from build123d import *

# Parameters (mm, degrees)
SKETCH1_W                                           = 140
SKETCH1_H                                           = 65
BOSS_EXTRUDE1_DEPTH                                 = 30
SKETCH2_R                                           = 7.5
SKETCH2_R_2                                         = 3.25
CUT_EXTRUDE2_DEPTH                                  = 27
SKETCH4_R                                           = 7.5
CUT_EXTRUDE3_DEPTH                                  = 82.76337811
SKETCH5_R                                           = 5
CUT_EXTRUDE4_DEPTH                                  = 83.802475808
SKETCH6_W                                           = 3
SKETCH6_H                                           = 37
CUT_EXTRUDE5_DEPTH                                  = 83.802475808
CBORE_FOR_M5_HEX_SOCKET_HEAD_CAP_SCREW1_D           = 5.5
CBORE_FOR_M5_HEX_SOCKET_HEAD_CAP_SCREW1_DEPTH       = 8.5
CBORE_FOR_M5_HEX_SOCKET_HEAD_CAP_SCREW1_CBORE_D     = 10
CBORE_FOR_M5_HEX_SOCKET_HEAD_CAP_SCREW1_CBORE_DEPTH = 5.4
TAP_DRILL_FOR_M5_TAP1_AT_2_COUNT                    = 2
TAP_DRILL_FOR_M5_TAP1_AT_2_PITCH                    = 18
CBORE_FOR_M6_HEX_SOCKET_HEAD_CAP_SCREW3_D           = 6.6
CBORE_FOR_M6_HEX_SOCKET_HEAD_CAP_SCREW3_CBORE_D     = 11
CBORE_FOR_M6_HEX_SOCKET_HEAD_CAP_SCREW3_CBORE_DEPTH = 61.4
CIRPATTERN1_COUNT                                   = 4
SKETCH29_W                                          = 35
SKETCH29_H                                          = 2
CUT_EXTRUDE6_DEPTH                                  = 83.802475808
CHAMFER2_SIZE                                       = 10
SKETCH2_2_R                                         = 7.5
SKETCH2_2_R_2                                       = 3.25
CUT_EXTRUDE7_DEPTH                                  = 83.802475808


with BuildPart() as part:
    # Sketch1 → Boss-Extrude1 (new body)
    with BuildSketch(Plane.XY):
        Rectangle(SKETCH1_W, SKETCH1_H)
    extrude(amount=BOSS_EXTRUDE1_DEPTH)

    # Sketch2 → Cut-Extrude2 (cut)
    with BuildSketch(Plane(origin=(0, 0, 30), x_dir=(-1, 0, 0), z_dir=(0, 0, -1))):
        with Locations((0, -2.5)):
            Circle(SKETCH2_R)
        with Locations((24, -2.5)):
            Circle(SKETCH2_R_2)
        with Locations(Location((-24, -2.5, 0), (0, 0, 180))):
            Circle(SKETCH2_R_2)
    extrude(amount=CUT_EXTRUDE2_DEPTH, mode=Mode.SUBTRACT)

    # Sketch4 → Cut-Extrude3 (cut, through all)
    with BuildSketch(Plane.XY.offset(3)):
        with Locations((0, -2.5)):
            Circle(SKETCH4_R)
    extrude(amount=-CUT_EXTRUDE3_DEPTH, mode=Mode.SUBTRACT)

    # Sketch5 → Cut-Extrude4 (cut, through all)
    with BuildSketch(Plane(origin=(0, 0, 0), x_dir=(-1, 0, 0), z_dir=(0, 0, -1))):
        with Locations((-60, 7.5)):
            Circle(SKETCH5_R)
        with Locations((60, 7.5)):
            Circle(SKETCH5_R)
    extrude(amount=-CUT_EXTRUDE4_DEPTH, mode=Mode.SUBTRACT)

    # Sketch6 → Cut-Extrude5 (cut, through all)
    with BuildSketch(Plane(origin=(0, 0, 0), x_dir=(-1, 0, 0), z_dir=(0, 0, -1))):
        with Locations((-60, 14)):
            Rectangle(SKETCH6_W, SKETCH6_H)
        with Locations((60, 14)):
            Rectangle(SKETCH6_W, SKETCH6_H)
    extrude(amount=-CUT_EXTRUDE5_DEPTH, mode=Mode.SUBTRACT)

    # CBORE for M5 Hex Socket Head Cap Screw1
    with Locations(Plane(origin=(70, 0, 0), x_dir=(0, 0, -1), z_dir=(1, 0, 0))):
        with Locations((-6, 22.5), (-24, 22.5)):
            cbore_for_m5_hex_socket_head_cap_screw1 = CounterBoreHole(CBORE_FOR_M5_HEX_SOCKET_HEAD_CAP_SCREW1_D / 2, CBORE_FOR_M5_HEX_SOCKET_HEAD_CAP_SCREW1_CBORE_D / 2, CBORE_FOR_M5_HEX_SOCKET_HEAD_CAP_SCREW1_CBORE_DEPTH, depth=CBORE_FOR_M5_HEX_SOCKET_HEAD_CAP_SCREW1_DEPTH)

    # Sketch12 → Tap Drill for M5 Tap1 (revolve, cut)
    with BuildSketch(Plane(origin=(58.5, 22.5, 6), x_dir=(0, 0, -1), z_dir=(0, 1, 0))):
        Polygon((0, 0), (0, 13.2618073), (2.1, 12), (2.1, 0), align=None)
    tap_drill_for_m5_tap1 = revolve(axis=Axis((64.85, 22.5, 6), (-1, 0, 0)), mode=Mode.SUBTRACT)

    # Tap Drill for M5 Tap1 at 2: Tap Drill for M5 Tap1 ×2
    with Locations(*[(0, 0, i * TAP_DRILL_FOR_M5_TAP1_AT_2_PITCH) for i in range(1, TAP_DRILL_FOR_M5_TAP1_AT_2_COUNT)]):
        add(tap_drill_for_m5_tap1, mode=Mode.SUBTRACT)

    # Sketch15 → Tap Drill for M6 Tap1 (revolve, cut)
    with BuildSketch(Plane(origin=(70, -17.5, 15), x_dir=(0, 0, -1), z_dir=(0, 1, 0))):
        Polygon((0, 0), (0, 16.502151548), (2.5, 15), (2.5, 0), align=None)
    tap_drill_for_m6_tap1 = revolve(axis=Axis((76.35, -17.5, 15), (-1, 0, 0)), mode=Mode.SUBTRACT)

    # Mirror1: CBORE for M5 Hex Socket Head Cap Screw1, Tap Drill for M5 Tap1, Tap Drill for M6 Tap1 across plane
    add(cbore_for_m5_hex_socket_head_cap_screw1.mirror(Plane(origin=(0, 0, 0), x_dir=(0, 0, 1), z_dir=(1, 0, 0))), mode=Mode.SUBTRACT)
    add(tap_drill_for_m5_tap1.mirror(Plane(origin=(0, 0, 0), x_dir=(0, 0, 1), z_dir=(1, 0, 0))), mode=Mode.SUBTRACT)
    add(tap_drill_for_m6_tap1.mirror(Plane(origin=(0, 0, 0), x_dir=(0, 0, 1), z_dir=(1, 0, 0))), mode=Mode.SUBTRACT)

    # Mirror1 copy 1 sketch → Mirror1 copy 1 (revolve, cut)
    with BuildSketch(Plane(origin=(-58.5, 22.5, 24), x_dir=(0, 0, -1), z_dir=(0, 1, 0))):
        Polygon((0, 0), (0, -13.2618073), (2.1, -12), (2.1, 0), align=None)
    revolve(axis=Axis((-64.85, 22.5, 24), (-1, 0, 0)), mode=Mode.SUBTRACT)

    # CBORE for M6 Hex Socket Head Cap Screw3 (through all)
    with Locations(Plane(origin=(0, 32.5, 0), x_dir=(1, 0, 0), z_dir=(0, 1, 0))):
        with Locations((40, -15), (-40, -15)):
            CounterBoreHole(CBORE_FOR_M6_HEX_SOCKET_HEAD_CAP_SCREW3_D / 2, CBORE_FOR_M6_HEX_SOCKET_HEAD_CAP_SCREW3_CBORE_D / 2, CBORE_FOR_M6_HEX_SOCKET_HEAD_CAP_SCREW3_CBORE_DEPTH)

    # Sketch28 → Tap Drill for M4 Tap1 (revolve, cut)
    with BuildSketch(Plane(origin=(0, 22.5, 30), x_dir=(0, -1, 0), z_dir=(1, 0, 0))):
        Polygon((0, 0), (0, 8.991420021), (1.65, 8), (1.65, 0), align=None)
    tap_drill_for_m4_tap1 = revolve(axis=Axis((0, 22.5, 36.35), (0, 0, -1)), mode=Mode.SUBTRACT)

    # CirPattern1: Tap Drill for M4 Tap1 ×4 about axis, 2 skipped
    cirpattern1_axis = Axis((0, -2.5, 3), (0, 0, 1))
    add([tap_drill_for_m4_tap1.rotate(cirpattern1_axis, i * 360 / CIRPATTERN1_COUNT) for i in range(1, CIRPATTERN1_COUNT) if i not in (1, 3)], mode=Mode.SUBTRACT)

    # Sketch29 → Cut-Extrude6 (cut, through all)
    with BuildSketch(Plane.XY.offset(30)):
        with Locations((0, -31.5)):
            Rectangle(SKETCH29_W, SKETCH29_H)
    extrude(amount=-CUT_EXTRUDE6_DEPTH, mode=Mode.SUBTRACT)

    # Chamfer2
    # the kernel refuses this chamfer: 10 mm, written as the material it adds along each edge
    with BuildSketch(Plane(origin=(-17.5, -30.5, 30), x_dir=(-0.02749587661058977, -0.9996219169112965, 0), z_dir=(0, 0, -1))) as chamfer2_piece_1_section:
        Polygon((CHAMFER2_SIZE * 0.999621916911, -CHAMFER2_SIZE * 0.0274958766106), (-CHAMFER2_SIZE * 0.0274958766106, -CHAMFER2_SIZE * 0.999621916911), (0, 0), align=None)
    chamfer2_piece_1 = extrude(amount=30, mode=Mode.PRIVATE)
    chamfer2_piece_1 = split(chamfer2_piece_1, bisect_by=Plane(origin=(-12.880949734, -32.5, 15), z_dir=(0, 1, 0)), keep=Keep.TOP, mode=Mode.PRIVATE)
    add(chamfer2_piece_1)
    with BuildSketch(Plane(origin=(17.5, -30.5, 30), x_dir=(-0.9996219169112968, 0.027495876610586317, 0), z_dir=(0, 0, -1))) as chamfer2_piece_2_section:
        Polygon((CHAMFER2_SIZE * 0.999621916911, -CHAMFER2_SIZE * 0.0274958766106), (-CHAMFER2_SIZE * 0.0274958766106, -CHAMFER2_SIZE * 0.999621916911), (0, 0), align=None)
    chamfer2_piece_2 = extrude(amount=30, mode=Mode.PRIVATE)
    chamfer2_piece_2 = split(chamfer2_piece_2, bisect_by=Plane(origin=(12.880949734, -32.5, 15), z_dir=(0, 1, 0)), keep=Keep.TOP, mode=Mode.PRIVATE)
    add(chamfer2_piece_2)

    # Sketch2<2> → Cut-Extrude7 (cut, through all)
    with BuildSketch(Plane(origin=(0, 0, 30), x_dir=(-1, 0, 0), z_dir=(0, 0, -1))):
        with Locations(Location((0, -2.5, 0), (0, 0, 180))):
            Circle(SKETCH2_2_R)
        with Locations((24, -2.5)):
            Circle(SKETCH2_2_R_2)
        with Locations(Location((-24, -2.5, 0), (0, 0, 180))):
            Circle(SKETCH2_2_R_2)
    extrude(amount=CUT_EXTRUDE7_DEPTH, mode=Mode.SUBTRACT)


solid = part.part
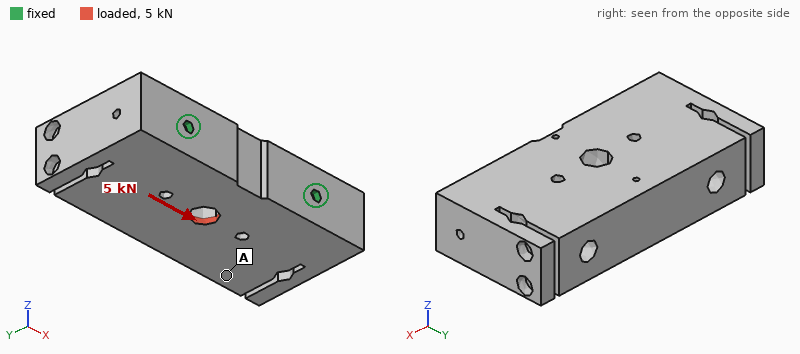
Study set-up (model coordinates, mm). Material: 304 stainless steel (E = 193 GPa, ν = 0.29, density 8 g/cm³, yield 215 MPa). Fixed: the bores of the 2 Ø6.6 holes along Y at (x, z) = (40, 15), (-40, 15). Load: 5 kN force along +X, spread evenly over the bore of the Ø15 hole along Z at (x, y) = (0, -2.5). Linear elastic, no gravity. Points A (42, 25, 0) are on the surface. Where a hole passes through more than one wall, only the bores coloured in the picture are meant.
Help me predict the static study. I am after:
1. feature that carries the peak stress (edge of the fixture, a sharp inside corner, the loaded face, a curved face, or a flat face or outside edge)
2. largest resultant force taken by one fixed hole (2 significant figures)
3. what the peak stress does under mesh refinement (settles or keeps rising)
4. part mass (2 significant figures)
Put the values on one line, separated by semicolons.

edge of the fixture; 3.2 kN; keeps rising; 1.9 kg
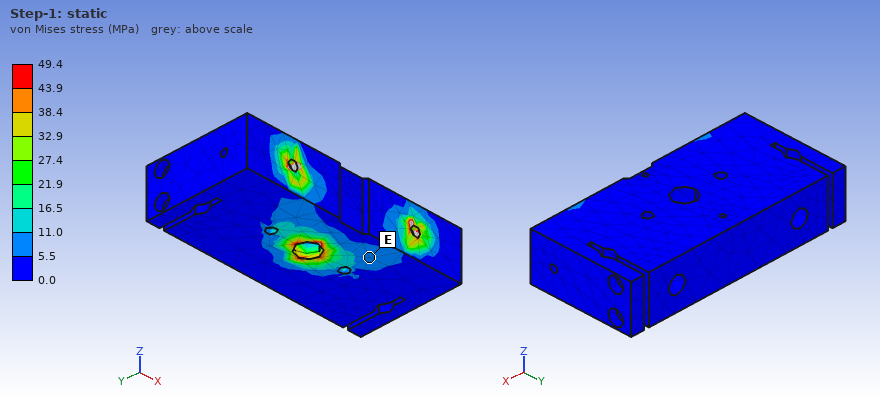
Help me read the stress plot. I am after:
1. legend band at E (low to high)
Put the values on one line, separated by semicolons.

5.5 to 11.0 MPa
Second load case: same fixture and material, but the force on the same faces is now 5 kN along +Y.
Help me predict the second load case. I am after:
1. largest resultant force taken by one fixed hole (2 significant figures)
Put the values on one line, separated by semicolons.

2.6 kN
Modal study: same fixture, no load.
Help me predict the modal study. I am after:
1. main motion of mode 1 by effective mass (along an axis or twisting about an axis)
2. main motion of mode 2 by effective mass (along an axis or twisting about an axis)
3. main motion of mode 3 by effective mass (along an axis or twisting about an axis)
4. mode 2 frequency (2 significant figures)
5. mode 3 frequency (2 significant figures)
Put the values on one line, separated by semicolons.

along Z; along X; twisting about Y; 3200 Hz; 3400 Hz
